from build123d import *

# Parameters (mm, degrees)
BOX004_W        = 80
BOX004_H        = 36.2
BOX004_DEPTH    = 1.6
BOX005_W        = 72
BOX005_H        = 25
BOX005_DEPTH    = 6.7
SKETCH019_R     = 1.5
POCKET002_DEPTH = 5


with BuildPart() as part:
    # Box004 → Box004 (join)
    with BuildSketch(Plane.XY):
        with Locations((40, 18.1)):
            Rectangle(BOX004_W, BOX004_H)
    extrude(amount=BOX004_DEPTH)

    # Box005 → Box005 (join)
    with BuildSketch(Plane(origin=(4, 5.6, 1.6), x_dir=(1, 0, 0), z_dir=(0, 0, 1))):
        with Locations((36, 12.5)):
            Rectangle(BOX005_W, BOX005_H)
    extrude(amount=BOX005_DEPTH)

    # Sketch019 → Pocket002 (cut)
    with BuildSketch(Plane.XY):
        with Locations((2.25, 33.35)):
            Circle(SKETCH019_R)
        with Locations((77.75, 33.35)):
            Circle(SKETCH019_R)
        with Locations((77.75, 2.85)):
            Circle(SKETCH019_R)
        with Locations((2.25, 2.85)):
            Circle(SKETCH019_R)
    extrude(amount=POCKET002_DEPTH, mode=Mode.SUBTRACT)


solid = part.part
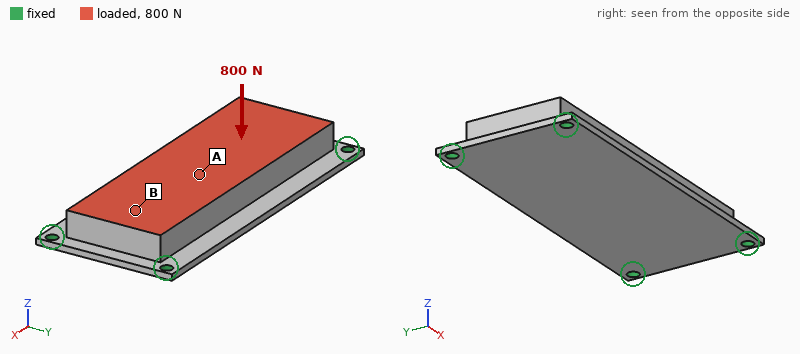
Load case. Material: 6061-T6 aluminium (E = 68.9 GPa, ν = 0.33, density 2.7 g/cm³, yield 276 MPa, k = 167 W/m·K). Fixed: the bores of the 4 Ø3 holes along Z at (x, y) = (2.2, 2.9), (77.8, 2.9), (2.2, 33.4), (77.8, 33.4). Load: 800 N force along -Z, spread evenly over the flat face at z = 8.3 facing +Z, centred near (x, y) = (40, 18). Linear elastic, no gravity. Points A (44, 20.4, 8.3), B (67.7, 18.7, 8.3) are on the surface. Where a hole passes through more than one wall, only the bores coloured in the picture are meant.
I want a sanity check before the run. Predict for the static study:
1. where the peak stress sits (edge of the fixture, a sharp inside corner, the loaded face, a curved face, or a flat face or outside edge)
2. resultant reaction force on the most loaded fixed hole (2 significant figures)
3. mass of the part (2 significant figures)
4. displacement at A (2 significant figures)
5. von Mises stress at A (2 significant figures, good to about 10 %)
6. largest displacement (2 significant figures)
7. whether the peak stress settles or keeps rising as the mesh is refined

edge of the fixture
380 N
45 g
38 µm
18 MPa
42 µm
keeps rising
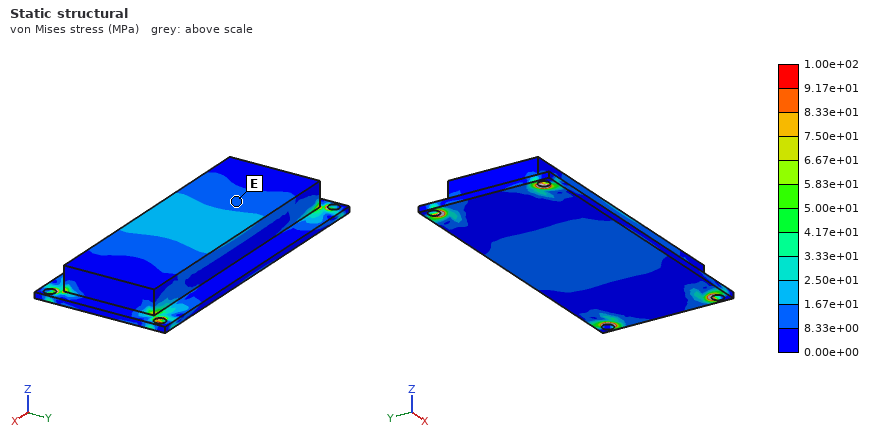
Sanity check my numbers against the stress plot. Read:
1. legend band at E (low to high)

8.33e+00 to 1.67e+01 MPa
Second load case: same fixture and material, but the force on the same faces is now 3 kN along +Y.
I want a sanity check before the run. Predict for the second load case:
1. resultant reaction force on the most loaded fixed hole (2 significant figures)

1.0 kN
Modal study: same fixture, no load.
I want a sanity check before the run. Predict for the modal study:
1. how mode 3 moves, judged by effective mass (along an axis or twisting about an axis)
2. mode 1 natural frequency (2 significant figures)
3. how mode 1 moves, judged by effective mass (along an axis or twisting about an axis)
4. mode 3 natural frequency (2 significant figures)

twisting about Y
3800 Hz
along Z
9200 Hz
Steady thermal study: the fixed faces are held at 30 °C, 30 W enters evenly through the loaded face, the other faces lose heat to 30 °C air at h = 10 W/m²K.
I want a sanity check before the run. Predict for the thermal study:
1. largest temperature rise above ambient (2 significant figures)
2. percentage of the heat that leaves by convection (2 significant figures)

22 K
3.3 %
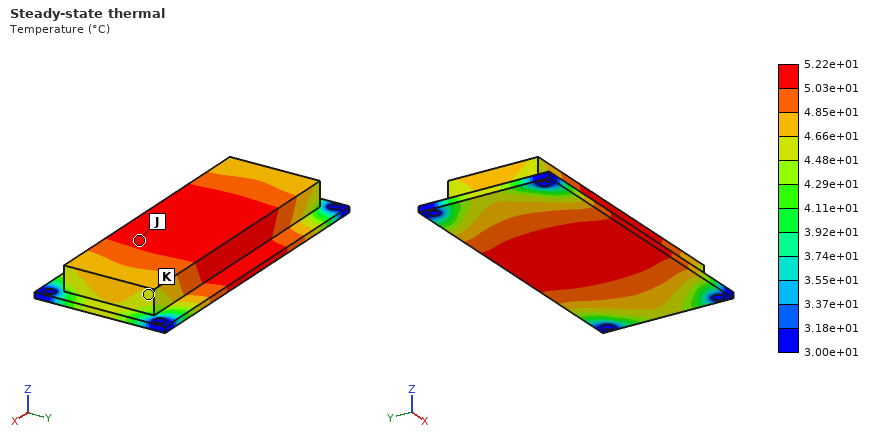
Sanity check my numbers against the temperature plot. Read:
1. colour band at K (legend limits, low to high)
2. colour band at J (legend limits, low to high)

4.48e+01 to 4.66e+01 °C
5.03e+01 to 5.22e+01 °C
